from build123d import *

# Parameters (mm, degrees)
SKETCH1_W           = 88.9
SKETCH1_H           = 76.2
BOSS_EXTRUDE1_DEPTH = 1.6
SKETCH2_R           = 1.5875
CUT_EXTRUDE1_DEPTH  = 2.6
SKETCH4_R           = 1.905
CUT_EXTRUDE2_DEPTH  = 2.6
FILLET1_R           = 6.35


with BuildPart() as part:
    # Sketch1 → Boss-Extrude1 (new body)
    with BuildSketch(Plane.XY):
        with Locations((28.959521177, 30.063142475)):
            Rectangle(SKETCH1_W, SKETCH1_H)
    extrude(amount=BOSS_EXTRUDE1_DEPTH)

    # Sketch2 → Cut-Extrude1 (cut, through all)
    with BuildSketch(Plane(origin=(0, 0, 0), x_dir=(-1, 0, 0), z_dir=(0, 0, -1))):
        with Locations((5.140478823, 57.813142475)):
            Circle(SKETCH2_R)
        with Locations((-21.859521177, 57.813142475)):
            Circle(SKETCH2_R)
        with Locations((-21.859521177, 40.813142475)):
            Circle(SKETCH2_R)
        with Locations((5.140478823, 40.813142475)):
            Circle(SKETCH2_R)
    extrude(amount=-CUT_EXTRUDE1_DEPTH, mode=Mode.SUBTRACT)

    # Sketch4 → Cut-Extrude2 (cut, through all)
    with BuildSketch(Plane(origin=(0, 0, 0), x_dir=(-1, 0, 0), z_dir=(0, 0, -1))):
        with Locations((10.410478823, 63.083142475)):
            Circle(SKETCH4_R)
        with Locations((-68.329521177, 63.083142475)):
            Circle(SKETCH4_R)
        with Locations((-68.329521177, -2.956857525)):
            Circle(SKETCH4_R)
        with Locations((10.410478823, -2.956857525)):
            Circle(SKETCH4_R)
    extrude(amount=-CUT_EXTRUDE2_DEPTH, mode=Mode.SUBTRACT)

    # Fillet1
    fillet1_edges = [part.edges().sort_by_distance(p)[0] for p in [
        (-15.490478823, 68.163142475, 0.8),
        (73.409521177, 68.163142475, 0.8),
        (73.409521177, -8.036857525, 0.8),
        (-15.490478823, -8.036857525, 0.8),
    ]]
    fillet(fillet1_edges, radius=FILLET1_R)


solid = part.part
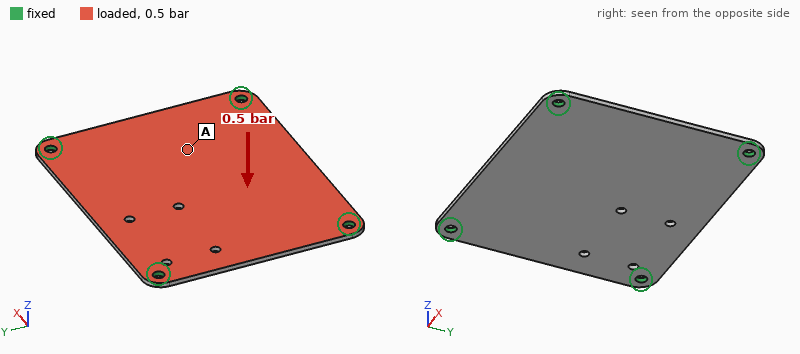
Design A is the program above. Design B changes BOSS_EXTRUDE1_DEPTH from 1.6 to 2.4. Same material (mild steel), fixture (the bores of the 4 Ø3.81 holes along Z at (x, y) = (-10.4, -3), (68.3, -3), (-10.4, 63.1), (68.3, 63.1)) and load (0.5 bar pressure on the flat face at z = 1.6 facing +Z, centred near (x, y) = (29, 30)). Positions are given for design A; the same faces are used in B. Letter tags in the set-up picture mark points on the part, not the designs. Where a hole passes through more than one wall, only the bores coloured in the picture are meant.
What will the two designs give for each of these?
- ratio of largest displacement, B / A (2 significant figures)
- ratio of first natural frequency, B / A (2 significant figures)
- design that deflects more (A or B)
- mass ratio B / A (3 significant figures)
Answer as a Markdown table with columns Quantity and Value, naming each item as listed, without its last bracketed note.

| Quantity | Value |
|---|---|
| ratio of largest displacement, B / A | 0.31 |
| ratio of first natural frequency, B / A | 1.5 |
| design that deflects more | A |
| mass ratio B / A | 1.50 |
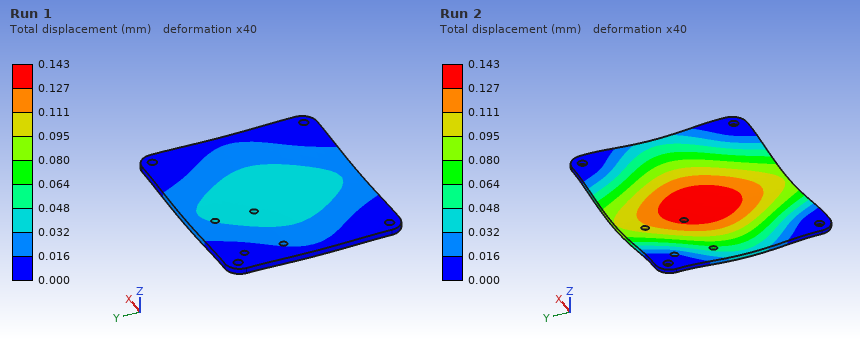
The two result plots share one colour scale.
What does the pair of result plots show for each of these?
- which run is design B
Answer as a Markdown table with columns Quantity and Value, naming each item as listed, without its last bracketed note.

| Quantity | Value |
|---|---|
| which run is design B | Run 1 |
